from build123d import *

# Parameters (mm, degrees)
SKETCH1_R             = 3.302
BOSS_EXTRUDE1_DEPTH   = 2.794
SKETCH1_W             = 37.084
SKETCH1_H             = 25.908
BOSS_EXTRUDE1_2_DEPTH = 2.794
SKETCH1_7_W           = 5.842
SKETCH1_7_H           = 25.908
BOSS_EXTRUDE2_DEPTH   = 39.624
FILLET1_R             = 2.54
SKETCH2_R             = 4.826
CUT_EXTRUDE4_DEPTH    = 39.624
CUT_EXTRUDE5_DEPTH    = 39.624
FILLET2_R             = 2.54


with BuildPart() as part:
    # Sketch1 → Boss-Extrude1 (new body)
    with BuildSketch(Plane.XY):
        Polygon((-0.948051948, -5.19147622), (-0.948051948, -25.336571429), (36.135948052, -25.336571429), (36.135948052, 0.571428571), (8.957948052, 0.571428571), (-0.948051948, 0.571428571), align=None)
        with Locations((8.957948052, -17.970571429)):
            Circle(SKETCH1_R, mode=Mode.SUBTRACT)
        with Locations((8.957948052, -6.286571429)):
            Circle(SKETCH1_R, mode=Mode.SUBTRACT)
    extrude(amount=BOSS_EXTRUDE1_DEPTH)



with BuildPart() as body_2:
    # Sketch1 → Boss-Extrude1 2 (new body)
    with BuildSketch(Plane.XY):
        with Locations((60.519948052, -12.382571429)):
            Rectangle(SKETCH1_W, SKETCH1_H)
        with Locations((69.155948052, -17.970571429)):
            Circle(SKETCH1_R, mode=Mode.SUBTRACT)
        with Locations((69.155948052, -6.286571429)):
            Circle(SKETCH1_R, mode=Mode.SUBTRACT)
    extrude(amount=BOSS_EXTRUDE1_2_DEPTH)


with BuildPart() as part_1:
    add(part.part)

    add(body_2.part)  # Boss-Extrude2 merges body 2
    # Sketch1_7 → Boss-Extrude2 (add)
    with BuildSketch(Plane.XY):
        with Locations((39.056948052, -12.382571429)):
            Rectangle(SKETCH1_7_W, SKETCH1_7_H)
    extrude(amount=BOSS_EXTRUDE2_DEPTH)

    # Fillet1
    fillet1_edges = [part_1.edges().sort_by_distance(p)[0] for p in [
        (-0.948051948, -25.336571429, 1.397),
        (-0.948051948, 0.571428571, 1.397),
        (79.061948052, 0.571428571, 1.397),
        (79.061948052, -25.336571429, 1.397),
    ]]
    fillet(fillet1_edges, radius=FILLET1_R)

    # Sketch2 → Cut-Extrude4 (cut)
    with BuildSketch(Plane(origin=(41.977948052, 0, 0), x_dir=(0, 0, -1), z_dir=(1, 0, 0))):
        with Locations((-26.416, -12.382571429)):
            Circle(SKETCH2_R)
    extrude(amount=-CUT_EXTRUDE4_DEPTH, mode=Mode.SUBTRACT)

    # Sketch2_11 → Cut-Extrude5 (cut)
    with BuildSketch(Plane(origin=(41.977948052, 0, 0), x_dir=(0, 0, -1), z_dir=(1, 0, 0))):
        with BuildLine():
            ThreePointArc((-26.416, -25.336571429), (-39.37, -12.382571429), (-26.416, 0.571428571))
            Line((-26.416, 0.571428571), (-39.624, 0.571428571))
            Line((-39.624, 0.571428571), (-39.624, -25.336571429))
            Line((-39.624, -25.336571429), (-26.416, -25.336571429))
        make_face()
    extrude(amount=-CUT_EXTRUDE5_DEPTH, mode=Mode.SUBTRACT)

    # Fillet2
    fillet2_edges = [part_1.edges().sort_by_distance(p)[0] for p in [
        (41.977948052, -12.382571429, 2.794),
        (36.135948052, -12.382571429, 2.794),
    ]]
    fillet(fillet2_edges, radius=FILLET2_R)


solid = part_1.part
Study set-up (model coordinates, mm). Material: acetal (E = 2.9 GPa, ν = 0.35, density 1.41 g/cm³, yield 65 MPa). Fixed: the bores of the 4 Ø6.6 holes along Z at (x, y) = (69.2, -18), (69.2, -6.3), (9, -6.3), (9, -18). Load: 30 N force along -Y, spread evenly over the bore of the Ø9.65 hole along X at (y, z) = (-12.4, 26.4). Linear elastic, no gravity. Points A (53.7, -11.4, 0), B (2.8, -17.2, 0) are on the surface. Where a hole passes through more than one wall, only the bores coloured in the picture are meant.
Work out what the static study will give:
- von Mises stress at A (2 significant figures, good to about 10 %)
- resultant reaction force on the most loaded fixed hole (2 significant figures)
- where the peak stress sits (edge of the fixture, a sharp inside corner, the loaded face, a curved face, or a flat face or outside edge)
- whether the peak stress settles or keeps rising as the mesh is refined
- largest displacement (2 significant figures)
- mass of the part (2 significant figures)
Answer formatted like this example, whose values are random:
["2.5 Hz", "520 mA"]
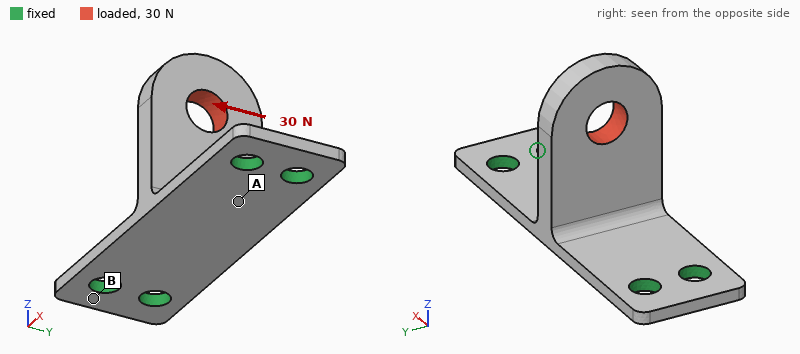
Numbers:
["7.0 MPa", "29 N", "edge of the fixture", "keeps rising", "1.0 mm", "14 g"]
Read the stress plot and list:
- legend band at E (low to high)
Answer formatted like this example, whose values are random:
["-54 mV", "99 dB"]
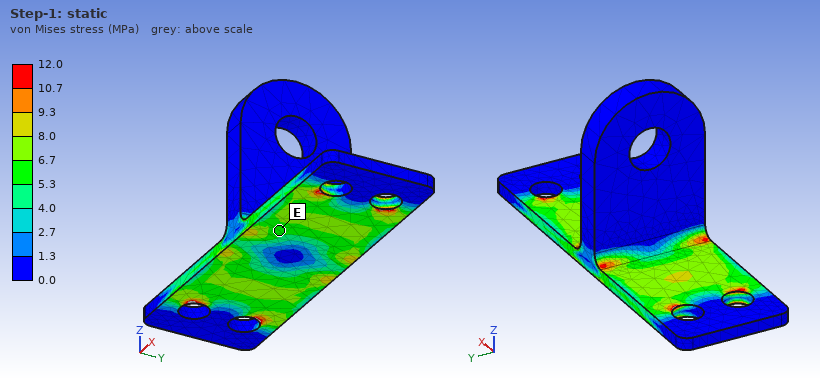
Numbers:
["5.3 to 6.7 MPa"]
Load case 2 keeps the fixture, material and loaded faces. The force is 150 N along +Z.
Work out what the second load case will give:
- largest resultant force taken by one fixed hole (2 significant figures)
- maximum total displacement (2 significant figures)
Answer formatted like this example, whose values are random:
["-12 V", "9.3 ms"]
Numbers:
["44 N", "0.69 mm"]
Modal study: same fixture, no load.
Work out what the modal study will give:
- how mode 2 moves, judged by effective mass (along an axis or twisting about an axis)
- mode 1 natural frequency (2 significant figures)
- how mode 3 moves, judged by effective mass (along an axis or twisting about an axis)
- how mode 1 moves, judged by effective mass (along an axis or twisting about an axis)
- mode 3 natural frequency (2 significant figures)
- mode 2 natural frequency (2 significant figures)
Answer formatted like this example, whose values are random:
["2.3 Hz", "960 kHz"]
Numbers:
["along X", "460 Hz", "along Z", "along Y", "780 Hz", "650 Hz"]
